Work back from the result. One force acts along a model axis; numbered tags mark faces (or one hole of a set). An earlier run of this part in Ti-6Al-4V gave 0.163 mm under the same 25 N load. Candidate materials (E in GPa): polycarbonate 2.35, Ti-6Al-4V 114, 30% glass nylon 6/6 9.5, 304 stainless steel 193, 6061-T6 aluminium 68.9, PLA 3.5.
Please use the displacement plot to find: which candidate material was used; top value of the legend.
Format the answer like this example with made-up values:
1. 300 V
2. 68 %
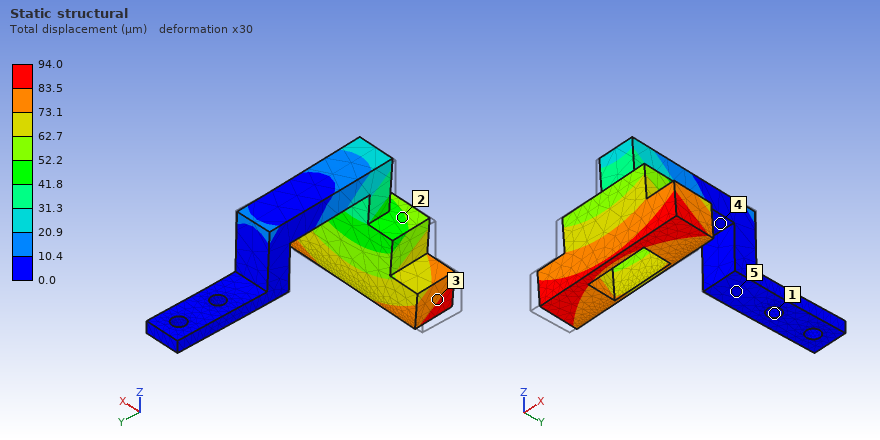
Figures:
1. 304 stainless steel
2. 94.0 µm
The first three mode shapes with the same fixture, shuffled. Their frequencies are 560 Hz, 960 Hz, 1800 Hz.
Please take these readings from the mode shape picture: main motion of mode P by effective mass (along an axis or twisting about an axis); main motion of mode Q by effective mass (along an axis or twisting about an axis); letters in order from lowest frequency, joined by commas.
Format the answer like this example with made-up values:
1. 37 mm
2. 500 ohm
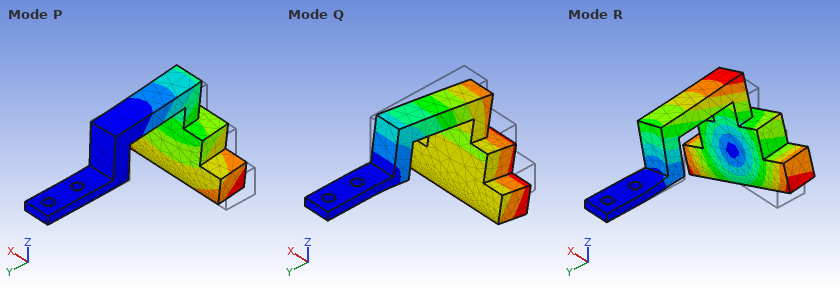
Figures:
1. along X
2. along Z
3. Q, P, R
